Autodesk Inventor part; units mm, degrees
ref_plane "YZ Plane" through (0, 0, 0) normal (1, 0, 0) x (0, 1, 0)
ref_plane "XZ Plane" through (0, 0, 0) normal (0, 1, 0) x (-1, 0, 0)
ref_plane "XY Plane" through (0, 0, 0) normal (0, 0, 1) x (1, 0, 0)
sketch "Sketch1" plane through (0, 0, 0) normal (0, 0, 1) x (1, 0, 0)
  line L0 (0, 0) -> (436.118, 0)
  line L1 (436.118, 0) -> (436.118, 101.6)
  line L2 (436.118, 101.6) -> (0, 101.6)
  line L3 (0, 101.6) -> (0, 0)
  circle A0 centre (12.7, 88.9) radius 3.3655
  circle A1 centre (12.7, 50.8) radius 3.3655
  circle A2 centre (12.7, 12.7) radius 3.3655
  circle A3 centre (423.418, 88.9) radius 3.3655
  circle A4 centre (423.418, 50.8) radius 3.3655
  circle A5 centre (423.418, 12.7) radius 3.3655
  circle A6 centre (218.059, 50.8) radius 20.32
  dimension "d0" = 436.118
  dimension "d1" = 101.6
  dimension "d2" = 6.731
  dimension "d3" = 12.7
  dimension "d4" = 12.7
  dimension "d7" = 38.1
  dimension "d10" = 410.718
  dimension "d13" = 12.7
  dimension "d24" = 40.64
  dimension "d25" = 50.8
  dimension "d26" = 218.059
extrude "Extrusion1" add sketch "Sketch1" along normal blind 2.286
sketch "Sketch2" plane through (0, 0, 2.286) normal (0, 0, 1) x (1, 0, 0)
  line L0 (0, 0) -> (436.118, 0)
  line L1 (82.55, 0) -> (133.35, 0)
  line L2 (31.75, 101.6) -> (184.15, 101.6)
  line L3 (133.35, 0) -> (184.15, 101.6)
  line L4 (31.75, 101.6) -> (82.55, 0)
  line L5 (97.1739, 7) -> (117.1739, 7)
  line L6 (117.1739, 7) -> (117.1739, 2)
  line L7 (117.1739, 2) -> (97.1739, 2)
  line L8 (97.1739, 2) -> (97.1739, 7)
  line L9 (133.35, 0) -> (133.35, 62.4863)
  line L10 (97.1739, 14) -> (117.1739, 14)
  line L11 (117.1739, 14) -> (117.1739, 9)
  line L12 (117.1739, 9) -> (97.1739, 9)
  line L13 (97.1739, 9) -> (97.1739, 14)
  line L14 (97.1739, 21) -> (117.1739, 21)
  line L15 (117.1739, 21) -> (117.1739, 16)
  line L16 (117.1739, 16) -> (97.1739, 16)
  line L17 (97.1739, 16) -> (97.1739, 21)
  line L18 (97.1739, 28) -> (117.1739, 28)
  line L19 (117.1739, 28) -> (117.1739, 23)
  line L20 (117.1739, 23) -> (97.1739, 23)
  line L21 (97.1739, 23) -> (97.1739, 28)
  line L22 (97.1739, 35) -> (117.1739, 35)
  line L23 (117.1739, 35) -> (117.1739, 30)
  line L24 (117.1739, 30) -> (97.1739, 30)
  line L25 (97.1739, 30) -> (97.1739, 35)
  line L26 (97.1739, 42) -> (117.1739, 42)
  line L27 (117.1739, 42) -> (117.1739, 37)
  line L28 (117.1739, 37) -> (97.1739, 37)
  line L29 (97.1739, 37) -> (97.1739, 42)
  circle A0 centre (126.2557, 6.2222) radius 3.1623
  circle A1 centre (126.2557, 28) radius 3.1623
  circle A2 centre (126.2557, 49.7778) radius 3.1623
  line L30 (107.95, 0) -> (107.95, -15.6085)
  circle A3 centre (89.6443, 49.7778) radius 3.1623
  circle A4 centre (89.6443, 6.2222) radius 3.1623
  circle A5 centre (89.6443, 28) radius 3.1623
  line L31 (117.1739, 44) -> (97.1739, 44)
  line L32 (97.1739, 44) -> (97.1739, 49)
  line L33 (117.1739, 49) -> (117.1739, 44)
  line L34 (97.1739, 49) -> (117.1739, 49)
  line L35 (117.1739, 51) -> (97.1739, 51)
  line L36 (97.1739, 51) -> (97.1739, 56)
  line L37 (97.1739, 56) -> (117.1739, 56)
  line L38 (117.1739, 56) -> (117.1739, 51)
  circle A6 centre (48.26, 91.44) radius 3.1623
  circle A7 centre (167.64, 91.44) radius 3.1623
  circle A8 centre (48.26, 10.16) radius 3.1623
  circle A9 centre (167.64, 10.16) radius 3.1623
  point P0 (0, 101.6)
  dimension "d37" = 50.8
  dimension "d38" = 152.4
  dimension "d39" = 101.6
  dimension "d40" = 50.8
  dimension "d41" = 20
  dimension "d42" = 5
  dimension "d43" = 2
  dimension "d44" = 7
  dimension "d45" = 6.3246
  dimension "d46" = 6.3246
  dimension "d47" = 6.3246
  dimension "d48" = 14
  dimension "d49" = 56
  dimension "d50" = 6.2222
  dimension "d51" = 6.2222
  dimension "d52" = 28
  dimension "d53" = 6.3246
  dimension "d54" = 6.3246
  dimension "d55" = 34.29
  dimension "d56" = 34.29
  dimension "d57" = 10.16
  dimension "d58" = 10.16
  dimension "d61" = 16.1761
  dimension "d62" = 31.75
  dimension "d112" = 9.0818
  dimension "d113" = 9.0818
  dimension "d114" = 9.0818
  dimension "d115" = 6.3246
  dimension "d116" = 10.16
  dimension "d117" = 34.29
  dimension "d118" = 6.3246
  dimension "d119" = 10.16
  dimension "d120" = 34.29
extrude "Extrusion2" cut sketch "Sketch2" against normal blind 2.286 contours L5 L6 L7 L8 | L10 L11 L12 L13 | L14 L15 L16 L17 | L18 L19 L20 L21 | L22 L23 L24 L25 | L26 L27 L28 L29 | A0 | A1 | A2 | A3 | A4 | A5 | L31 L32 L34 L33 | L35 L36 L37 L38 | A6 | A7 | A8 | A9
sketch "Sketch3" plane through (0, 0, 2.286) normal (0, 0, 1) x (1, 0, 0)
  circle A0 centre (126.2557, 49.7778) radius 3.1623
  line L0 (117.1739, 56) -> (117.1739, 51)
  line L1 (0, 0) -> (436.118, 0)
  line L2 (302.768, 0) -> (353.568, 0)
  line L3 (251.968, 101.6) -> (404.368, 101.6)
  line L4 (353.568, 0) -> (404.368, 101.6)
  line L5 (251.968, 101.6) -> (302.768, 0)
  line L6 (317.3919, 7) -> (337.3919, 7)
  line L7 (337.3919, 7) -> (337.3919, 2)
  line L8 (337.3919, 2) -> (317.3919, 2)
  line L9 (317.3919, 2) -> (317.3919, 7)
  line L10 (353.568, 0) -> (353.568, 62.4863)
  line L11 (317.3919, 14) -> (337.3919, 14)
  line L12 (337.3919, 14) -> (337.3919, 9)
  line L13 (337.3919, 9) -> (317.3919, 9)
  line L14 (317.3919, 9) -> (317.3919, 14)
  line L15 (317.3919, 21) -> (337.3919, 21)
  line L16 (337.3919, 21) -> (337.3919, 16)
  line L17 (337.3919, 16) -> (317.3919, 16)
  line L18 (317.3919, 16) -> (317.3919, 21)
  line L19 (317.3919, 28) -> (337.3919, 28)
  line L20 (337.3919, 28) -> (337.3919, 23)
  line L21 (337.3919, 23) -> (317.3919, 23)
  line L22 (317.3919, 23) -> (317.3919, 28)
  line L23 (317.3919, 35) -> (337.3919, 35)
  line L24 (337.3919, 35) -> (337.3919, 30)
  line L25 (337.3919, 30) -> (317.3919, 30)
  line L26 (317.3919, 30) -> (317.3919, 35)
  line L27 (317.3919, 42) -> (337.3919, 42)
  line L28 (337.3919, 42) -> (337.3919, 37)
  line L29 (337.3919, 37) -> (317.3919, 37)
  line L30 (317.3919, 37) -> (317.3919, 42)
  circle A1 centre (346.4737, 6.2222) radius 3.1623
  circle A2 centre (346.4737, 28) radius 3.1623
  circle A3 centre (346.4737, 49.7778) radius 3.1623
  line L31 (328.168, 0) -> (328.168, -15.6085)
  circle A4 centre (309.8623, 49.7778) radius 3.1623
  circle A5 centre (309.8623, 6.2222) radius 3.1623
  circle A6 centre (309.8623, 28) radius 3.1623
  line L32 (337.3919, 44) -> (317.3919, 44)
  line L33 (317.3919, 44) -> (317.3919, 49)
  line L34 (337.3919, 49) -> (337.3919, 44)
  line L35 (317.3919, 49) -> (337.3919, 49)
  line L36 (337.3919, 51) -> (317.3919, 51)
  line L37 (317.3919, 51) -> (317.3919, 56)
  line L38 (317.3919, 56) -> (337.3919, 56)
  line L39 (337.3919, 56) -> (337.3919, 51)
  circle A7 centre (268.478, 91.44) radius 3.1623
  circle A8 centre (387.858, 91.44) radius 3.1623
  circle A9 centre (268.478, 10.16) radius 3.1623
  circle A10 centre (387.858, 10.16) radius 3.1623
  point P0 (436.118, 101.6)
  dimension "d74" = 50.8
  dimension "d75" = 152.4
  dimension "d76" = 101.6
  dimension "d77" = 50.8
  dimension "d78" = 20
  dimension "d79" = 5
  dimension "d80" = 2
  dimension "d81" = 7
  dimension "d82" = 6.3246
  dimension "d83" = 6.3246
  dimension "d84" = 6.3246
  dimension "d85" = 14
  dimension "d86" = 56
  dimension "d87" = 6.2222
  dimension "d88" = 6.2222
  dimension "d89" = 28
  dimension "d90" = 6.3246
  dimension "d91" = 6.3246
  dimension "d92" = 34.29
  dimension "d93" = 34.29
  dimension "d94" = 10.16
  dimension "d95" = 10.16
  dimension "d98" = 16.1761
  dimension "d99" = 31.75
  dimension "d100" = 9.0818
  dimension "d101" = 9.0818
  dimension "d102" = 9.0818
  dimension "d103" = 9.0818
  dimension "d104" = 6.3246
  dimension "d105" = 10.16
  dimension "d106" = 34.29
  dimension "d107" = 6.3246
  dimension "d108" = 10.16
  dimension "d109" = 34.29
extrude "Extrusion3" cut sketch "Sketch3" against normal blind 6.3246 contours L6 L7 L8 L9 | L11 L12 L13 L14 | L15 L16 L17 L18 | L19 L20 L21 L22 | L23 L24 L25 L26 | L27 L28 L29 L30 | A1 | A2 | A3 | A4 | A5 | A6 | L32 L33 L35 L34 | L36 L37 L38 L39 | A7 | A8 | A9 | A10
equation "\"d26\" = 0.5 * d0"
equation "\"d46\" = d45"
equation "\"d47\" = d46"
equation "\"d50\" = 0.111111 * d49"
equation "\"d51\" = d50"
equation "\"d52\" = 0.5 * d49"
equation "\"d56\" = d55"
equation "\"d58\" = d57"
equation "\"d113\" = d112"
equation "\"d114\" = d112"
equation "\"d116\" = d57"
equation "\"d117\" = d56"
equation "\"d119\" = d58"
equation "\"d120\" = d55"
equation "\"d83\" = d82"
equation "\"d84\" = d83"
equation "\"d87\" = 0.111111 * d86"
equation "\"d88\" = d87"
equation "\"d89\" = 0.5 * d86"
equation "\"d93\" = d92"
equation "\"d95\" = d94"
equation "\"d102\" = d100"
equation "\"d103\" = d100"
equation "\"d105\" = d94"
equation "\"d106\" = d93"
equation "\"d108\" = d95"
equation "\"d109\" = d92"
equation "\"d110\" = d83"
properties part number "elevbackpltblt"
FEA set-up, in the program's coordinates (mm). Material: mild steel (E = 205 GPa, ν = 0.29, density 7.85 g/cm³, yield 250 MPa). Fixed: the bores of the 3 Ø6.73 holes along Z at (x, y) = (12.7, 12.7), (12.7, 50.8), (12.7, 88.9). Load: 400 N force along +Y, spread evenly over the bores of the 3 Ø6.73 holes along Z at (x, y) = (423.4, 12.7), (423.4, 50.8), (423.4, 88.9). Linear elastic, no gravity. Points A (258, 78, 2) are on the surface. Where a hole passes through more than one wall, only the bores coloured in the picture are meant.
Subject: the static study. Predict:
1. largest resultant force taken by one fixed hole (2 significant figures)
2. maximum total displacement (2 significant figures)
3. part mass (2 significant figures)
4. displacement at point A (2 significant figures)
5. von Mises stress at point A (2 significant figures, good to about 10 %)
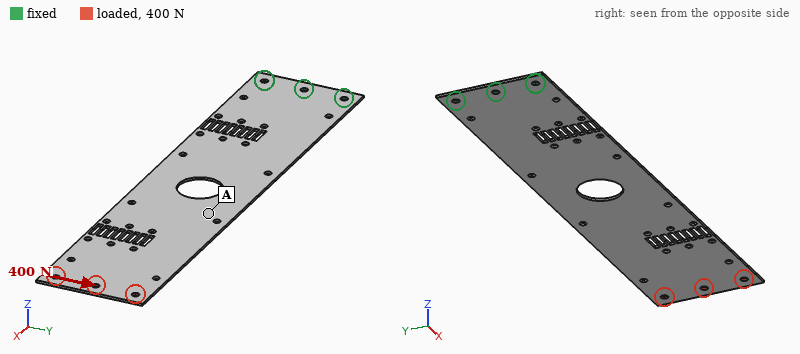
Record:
2.1 kN
0.31 mm
730 g
0.13 mm
11 MPa
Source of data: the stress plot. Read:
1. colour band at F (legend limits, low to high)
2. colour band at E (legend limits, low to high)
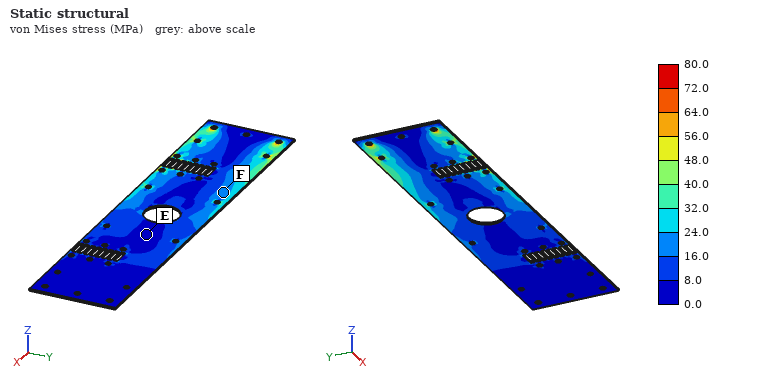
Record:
16.0 to 24.0 MPa
0.0 to 8.0 MPa
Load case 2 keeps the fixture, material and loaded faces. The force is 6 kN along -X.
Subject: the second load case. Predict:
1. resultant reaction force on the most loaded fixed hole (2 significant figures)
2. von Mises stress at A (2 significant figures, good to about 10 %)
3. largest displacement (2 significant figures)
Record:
2.1 kN
34 MPa
95 µm
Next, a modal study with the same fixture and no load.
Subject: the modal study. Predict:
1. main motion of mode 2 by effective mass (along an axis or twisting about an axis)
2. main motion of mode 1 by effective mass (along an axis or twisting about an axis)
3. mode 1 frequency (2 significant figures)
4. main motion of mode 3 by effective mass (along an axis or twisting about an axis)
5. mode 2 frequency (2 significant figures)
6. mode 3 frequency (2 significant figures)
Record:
along Z
along Z
10 Hz
twisting about X
65 Hz
86 Hz
